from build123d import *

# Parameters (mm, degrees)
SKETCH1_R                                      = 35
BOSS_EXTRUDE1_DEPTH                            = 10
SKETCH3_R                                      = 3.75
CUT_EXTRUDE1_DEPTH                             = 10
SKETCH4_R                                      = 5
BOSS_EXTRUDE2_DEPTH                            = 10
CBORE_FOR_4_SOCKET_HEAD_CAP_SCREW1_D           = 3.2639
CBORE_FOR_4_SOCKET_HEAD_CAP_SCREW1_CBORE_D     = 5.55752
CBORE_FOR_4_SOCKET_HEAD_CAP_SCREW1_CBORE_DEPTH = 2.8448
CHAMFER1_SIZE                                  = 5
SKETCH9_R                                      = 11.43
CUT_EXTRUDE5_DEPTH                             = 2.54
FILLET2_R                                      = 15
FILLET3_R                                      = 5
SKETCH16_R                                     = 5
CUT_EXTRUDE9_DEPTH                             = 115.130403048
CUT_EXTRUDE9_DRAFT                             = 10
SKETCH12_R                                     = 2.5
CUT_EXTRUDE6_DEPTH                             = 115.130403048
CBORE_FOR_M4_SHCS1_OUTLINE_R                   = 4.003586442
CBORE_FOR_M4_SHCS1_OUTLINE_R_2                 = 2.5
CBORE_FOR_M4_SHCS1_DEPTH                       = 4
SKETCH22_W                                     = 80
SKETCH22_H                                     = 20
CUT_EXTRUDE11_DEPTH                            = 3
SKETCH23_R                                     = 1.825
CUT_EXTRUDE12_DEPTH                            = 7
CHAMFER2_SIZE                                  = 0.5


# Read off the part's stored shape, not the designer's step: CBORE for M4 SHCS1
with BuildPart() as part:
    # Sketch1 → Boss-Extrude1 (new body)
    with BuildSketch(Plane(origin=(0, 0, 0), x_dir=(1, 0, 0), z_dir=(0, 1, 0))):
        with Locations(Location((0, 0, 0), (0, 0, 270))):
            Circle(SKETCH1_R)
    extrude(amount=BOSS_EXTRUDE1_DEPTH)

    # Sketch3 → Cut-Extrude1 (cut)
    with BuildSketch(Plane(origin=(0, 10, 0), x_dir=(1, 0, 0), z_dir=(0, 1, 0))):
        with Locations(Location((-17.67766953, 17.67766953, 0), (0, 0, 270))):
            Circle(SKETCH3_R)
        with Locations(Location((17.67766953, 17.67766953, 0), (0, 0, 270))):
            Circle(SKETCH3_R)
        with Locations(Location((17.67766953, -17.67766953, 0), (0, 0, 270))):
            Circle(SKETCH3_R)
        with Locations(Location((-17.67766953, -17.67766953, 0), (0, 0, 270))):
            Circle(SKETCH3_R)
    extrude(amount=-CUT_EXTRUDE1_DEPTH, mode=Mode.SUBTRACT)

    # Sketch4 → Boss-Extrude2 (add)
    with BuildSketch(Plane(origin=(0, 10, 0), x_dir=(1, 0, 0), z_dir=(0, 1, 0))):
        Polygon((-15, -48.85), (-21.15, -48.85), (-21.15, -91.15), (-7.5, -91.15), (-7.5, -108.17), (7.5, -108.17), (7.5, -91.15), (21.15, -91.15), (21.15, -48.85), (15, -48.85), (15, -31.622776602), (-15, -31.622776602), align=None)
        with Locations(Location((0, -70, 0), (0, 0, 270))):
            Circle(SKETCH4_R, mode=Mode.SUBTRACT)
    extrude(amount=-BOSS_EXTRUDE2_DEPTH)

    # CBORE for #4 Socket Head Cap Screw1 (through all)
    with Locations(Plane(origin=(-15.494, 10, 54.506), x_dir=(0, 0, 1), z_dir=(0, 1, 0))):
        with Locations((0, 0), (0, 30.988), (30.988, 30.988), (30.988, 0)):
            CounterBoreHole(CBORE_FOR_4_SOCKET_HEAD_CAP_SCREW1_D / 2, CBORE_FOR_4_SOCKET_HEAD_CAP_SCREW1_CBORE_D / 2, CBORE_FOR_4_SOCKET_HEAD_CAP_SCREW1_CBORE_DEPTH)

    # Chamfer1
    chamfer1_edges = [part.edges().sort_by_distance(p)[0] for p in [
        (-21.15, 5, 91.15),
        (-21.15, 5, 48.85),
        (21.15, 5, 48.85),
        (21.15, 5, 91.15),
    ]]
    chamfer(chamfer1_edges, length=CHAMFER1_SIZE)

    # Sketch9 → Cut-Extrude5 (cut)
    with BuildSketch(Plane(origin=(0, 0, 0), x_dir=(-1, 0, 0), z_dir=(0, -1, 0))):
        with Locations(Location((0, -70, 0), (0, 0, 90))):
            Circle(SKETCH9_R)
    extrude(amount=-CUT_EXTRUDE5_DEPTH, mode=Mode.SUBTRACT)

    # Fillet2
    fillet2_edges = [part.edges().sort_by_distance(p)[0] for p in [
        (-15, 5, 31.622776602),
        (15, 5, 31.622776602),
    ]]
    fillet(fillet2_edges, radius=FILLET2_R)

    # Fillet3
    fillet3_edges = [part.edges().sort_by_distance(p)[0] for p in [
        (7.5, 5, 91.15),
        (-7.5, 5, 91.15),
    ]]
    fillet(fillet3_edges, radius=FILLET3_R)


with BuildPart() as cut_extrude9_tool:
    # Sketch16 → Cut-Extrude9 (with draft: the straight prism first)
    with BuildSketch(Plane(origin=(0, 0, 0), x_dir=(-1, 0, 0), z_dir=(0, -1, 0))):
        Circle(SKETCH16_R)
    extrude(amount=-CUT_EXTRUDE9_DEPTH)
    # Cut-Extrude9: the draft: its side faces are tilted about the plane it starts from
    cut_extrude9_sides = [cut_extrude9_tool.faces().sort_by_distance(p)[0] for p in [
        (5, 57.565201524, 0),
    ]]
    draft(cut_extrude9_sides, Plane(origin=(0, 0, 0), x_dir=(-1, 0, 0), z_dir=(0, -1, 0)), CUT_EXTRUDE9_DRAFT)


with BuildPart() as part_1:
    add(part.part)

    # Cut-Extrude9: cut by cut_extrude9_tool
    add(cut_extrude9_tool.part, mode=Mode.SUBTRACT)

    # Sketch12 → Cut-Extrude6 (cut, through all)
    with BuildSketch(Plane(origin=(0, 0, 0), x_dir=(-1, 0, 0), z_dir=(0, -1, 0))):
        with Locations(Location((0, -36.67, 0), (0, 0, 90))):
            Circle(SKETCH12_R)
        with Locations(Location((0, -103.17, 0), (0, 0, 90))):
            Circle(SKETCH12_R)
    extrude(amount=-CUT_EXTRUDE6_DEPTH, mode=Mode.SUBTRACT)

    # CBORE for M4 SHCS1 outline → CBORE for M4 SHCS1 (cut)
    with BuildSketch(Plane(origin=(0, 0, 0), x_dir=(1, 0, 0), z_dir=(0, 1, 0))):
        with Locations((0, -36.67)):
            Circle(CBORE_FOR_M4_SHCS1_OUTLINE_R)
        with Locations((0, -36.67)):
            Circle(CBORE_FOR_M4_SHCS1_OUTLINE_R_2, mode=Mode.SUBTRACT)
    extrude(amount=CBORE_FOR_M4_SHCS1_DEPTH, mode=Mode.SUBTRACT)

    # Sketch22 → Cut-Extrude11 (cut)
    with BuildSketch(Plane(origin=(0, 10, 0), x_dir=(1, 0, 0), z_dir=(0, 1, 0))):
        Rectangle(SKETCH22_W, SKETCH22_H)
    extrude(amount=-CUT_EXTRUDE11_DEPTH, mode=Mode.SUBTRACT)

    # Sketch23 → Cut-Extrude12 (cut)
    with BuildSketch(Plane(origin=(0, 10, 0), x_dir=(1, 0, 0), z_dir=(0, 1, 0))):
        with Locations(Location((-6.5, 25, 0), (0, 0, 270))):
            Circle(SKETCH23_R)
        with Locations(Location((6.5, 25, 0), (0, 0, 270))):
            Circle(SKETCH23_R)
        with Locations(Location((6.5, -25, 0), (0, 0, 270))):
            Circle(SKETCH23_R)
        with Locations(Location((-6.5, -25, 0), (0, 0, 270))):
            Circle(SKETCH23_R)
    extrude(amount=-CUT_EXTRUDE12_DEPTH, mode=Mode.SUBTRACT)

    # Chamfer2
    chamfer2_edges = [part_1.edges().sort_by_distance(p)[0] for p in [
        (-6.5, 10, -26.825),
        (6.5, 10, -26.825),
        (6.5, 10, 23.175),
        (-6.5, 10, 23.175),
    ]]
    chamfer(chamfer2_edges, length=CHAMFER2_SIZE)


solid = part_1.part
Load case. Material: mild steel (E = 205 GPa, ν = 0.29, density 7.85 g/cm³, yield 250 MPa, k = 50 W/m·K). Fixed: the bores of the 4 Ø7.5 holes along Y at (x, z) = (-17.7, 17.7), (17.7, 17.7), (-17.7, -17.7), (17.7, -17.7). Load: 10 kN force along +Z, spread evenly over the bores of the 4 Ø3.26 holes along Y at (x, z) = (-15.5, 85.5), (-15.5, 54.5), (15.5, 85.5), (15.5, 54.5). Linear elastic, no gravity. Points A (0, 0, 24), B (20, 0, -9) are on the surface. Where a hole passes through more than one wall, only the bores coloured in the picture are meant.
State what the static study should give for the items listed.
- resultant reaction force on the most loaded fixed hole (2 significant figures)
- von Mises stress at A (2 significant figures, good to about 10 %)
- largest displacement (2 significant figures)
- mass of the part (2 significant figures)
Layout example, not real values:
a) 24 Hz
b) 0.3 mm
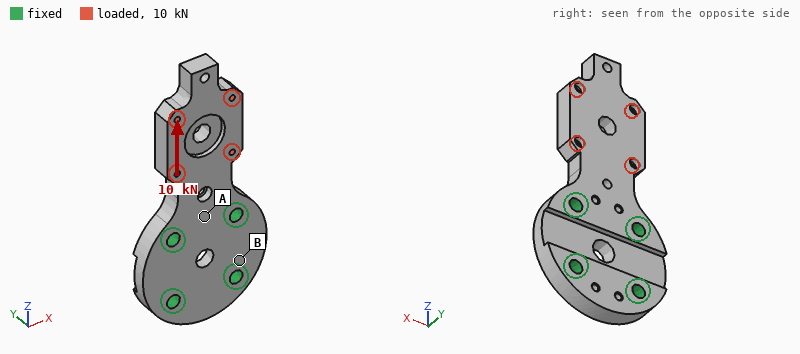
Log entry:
a) 4.8 kN
b) 26 MPa
c) 97 µm
d) 420 g
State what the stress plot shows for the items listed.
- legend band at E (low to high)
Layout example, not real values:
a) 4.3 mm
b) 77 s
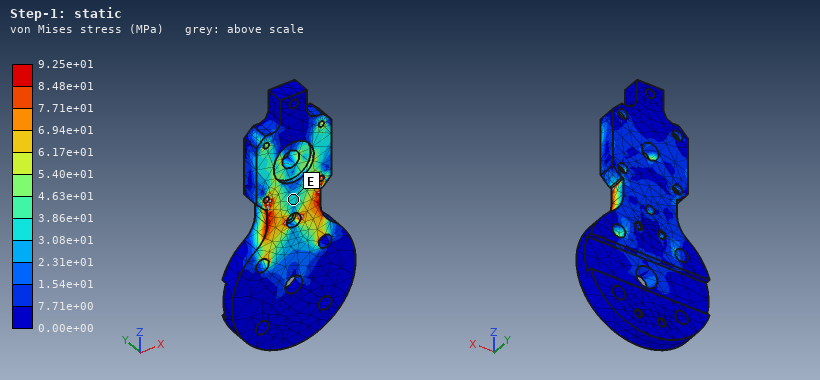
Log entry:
a) 3.08e+01 to 3.86e+01 MPa
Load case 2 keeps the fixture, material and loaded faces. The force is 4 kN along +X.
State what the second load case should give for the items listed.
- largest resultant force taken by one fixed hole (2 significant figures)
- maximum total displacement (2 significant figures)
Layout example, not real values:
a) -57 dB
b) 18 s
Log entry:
a) 5.8 kN
b) 69 µm
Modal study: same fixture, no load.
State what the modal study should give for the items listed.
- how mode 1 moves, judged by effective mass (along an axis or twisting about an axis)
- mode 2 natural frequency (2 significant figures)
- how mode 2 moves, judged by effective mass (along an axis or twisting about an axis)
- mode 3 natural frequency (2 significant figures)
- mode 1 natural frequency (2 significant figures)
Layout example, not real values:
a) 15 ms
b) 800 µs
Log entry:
a) along Y
b) 3800 Hz
c) along X
d) 4600 Hz
e) 1200 Hz
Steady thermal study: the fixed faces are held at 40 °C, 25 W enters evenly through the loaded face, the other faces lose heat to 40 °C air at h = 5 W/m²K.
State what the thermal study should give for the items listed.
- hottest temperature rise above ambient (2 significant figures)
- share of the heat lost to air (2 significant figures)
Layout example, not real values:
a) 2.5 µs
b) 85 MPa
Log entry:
a) 81 K
b) 9.6 %
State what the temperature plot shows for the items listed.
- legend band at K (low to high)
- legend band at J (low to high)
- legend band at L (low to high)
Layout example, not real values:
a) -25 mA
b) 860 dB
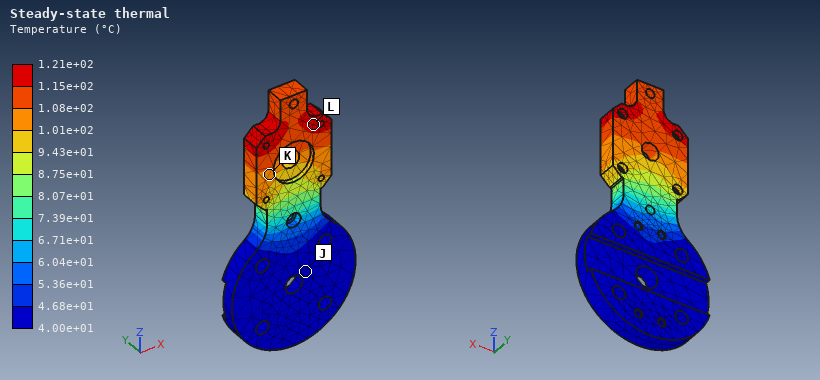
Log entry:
a) 1.01e+02 to 1.08e+02 °C
b) 4.00e+01 to 4.68e+01 °C
c) 1.15e+02 to 1.21e+02 °C
